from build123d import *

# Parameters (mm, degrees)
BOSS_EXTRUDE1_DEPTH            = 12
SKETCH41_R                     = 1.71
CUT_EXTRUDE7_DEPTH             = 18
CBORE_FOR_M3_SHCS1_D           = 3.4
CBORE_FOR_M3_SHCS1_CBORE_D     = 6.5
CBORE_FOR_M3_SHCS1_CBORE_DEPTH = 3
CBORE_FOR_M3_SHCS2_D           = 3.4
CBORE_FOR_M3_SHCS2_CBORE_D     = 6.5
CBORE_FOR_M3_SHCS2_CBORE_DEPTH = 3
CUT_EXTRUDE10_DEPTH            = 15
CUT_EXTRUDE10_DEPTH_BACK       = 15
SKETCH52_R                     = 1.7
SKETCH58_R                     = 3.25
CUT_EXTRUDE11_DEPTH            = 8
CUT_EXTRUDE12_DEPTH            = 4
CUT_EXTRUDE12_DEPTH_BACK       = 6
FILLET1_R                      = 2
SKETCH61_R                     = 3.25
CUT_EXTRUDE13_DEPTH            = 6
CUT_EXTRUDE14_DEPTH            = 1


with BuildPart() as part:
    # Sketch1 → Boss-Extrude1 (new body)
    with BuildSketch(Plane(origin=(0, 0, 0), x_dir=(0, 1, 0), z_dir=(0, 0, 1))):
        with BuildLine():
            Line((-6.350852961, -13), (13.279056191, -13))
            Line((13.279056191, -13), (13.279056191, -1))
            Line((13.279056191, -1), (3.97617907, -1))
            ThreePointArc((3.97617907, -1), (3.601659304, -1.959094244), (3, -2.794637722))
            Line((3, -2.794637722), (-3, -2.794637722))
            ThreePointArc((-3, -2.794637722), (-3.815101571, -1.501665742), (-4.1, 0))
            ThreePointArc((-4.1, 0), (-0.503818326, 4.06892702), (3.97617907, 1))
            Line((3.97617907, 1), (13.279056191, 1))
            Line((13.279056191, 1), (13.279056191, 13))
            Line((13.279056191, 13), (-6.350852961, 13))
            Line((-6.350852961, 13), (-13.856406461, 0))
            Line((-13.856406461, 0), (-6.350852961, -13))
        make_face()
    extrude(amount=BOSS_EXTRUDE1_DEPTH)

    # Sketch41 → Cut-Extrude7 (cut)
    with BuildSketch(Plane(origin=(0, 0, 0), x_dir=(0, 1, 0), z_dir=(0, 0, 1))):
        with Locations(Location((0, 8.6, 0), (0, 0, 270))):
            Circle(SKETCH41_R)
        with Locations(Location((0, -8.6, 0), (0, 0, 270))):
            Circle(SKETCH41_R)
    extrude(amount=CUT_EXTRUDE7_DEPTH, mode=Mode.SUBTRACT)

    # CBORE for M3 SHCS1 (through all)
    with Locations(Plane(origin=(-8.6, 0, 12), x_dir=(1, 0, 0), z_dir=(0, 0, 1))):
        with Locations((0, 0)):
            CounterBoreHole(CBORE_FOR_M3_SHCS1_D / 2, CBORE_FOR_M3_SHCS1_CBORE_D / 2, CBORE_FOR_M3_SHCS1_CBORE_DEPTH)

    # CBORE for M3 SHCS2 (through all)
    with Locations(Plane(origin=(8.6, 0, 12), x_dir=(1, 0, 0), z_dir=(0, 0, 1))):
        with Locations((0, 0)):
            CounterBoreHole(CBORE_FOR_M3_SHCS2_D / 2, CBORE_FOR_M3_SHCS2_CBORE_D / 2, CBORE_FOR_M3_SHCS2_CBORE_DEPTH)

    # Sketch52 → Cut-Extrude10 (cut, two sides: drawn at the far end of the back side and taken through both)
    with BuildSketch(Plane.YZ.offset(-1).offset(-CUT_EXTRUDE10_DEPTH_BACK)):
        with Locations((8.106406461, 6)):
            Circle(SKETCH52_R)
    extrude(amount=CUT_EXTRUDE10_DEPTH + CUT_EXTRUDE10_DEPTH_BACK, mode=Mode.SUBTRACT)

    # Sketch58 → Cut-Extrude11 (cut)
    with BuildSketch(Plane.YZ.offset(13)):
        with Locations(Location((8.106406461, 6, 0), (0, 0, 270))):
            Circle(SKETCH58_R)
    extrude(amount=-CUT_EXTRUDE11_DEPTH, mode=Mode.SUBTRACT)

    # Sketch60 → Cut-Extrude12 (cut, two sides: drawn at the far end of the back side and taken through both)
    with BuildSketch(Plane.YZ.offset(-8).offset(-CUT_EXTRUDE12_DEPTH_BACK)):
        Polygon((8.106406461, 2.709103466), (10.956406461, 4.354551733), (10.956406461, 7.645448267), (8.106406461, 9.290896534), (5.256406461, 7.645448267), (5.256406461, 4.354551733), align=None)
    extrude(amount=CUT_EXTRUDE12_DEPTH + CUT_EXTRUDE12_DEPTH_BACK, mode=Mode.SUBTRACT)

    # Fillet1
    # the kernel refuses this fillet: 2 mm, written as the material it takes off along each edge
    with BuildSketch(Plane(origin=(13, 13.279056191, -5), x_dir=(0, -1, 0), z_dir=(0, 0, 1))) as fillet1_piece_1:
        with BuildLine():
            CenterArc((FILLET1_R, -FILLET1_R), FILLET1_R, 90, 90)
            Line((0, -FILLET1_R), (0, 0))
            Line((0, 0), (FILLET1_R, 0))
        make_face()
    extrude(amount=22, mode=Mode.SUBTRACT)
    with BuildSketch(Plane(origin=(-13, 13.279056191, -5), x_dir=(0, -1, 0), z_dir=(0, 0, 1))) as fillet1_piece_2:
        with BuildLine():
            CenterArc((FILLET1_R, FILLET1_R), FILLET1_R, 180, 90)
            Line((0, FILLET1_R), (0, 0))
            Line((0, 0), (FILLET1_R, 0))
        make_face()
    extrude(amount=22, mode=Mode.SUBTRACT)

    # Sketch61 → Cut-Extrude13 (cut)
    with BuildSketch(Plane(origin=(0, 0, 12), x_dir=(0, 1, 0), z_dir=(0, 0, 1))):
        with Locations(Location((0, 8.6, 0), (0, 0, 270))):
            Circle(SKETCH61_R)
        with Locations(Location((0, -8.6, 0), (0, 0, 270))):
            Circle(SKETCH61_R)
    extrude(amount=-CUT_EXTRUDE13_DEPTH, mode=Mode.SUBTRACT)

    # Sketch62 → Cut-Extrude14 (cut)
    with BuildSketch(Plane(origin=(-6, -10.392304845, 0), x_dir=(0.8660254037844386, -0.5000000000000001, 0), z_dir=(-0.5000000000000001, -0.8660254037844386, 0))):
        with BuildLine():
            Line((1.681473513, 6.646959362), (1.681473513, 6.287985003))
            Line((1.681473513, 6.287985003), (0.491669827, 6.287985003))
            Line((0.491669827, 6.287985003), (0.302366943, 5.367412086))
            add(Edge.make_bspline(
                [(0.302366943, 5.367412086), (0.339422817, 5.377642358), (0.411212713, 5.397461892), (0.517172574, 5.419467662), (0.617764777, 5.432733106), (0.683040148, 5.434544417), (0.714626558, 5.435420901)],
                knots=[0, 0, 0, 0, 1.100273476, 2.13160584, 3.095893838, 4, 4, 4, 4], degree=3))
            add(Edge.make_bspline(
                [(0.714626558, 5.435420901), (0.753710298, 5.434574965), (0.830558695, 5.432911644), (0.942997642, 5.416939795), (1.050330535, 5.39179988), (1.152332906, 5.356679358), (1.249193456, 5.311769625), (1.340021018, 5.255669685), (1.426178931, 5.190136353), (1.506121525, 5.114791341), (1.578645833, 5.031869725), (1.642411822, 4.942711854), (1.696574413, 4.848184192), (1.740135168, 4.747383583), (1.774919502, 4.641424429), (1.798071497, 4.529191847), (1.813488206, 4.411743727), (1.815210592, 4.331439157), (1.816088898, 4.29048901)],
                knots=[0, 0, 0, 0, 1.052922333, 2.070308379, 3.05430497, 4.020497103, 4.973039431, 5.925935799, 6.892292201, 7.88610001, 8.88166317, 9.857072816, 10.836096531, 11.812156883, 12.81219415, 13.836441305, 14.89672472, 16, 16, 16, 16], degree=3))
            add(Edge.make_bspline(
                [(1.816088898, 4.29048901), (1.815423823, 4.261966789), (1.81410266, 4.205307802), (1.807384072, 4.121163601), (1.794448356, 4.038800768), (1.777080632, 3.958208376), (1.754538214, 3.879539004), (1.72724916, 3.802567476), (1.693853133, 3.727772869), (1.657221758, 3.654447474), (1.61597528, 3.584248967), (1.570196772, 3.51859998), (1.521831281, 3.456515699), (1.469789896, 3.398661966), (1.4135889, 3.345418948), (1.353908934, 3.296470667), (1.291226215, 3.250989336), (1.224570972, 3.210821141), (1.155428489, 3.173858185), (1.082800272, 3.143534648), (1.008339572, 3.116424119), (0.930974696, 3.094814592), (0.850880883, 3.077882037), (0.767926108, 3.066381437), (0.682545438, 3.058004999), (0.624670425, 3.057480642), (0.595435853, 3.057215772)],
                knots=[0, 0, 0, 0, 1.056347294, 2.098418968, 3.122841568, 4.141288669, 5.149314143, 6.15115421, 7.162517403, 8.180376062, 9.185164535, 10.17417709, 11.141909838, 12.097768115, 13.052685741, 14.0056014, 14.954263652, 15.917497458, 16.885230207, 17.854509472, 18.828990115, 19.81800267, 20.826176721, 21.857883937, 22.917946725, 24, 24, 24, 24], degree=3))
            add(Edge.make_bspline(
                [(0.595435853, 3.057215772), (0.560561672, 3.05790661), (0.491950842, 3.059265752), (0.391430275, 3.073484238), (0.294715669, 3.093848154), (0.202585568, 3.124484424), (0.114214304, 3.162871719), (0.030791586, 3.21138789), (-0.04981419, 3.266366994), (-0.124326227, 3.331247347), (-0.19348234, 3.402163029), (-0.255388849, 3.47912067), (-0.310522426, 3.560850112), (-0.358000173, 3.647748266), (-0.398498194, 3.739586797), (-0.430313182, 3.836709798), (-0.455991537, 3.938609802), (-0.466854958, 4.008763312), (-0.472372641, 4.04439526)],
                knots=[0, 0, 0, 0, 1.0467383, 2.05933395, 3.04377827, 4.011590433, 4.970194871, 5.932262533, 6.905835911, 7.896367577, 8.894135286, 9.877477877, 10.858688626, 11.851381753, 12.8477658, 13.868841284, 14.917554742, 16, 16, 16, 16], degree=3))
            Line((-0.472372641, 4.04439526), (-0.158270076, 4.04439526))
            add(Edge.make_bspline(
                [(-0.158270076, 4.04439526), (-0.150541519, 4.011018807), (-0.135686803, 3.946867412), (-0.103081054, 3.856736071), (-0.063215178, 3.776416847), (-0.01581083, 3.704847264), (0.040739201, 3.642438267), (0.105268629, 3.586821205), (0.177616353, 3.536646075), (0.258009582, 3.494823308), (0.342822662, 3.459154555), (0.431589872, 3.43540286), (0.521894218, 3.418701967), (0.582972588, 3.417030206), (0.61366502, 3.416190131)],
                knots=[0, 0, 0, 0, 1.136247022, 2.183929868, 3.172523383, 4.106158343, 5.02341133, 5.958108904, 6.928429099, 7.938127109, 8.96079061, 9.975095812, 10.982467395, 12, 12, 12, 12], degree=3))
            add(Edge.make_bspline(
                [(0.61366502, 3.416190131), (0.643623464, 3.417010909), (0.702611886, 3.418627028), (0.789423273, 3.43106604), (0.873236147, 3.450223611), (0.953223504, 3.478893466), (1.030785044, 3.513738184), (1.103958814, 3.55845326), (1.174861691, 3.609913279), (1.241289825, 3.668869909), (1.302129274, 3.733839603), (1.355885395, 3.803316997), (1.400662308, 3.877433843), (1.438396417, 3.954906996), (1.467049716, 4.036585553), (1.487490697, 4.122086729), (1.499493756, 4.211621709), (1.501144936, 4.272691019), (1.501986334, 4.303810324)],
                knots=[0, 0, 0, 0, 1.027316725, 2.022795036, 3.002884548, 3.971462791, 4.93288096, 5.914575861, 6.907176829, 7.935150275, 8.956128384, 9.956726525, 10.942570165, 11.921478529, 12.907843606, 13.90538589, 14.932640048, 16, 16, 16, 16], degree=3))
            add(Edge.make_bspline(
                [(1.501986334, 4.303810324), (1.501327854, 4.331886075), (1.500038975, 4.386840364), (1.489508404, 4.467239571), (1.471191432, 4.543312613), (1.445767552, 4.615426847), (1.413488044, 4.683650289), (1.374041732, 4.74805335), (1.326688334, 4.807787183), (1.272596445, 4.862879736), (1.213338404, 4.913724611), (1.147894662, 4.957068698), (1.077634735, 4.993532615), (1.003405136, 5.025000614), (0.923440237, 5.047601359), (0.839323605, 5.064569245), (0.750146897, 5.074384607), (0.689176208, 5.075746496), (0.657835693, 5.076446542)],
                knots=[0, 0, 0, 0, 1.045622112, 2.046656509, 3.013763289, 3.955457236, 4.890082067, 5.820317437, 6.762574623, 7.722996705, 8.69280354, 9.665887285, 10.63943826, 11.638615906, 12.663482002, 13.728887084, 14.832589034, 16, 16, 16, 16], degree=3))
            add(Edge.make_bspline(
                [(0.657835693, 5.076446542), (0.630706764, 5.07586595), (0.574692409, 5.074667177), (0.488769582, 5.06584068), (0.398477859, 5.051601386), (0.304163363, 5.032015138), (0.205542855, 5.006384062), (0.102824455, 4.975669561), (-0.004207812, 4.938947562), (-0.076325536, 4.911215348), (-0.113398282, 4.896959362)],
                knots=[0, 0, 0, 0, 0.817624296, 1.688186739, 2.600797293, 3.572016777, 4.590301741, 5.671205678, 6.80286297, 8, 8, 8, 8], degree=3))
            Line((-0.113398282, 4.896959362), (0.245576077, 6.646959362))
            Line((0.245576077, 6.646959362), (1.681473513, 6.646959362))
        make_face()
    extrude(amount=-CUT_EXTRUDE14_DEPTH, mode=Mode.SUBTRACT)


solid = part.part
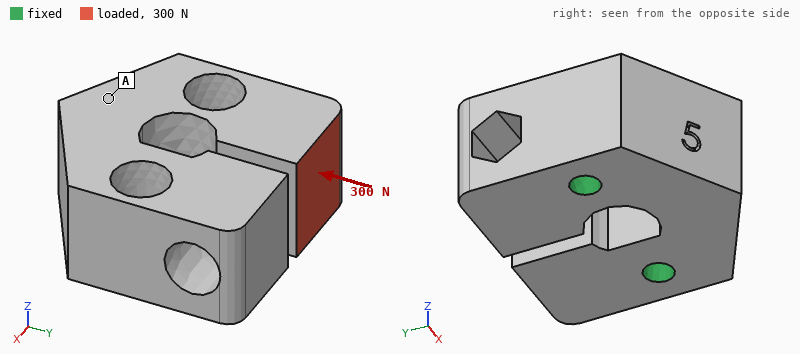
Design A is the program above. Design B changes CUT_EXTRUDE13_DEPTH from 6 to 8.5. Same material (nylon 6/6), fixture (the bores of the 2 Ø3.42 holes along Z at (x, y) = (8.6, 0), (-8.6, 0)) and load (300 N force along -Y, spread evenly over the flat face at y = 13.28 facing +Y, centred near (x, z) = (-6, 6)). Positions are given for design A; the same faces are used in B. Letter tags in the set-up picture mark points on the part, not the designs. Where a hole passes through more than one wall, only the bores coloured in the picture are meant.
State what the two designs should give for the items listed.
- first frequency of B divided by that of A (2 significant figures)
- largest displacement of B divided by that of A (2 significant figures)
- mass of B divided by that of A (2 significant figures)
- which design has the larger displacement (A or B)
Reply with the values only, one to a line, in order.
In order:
0.59
2.0
0.98
B
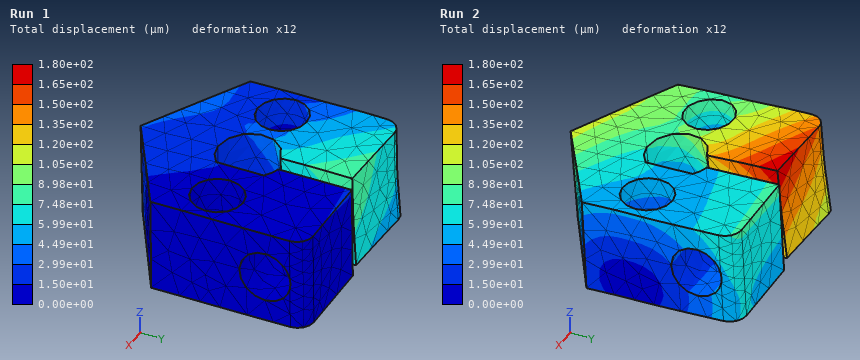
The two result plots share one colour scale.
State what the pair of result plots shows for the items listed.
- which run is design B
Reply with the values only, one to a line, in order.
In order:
Run 2
